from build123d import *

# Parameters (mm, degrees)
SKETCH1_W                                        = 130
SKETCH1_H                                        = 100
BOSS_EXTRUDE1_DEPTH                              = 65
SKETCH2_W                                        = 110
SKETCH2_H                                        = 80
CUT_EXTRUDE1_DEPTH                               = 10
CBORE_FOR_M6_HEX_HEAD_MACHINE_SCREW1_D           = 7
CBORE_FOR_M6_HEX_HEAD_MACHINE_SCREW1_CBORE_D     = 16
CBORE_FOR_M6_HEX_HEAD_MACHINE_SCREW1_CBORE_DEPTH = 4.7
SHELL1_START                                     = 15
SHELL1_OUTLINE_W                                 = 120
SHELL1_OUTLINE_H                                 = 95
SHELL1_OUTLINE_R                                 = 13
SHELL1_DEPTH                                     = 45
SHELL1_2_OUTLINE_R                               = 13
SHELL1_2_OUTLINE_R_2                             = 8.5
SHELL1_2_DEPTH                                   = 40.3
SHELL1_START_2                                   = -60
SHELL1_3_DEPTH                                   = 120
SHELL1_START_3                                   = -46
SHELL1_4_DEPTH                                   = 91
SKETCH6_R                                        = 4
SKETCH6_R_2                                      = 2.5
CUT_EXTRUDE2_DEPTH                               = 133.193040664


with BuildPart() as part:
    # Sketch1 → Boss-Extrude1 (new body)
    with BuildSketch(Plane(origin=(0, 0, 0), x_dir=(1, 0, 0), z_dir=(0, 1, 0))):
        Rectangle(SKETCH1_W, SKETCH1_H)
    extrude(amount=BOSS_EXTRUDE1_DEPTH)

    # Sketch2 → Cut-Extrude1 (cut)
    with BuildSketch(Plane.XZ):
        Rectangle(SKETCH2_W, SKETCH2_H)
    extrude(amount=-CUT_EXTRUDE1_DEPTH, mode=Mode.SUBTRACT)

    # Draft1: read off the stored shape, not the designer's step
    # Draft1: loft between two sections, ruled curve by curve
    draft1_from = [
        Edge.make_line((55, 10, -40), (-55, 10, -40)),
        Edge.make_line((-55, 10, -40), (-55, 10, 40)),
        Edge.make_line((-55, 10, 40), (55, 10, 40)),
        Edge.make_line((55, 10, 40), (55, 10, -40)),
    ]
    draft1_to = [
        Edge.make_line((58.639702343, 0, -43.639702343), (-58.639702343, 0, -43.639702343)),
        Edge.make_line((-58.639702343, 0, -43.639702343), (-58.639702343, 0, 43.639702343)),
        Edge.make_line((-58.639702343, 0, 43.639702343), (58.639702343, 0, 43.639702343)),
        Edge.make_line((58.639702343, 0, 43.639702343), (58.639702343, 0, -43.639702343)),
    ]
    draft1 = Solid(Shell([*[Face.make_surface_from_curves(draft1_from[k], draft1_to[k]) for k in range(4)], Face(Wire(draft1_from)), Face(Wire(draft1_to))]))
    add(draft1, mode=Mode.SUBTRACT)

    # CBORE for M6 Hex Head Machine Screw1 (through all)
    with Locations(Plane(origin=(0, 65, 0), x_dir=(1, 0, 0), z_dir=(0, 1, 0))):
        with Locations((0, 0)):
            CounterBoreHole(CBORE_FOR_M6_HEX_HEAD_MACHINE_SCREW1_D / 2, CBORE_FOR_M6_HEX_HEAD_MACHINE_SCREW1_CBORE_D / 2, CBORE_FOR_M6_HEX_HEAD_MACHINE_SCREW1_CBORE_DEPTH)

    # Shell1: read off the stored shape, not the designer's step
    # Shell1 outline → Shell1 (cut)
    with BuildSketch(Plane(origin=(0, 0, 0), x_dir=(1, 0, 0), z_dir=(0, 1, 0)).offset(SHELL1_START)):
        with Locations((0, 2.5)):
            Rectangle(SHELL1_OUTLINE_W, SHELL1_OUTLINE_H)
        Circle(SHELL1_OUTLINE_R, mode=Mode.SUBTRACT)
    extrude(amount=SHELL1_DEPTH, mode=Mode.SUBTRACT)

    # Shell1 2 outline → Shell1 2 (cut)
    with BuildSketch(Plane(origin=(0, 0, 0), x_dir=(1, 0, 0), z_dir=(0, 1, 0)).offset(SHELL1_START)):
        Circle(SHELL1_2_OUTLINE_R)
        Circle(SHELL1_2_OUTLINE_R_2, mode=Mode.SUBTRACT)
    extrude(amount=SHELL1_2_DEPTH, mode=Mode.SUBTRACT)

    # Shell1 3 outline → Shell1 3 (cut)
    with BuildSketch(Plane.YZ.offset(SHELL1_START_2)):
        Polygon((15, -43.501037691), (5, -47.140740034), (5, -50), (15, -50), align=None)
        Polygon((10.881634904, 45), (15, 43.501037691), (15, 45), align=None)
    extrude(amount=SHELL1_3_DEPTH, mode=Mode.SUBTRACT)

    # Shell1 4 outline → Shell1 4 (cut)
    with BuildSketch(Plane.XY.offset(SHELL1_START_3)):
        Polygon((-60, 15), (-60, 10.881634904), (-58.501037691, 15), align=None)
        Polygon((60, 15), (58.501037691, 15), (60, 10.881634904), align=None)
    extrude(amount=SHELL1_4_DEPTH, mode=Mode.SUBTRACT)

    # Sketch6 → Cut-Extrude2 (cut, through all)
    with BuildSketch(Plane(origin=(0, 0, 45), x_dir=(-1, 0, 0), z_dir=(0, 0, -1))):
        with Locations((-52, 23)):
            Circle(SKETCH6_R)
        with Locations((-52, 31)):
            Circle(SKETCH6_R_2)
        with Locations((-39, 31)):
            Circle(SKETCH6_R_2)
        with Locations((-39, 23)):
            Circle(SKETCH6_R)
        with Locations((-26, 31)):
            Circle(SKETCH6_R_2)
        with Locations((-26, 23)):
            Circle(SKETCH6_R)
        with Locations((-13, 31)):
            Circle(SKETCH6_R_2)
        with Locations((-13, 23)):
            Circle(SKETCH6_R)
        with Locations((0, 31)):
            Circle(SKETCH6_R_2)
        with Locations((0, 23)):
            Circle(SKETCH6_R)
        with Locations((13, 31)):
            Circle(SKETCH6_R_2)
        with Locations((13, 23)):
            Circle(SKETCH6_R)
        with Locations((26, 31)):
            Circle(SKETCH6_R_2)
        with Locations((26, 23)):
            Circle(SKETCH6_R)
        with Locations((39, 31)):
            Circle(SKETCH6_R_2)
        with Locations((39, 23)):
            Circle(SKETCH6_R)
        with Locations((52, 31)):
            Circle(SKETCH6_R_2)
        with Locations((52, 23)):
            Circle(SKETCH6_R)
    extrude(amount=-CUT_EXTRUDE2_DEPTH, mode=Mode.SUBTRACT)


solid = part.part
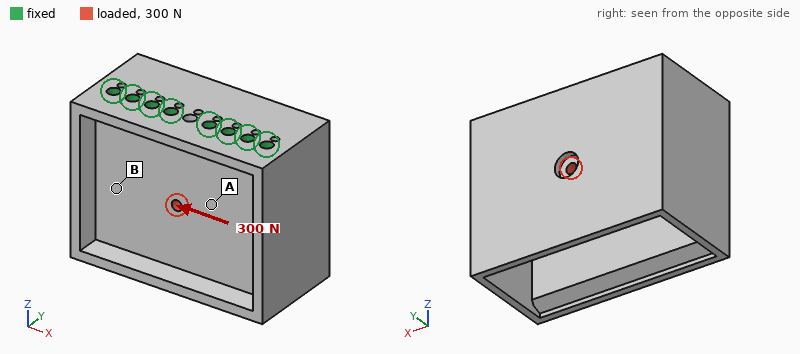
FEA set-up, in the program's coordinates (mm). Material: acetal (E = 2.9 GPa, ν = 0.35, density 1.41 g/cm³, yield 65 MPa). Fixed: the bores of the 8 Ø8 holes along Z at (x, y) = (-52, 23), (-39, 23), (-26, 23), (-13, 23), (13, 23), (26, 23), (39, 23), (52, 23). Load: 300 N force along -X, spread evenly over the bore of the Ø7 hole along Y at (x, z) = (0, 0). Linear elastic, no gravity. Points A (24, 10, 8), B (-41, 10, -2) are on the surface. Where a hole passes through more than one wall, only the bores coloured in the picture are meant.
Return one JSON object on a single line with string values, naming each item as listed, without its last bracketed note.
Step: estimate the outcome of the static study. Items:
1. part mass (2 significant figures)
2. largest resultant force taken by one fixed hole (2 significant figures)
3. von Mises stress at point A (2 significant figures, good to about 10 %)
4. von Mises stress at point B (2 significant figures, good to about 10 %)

{"part mass": "330 g", "largest resultant force taken by one fixed hole": "120 N", "von Mises stress at point A": "0.96 MPa", "von Mises stress at point B": "0.39 MPa"}
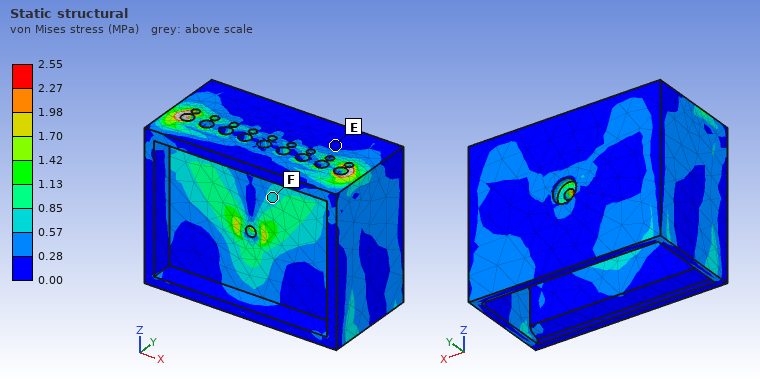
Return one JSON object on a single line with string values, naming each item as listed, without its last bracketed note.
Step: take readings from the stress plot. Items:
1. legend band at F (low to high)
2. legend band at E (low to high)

{"legend band at F": "0.57 to 0.85 MPa", "legend band at E": "0.00 to 0.28 MPa"}
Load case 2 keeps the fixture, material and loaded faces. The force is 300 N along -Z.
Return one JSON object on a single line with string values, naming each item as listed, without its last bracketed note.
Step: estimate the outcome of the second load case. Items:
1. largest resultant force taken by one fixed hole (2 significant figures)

{"largest resultant force taken by one fixed hole": "130 N"}
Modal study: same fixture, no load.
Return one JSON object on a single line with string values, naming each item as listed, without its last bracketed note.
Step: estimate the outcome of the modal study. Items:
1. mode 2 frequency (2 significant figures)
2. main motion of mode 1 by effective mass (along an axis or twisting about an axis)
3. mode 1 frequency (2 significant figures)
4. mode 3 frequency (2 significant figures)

{"mode 2 frequency": "400 Hz", "main motion of mode 1 by effective mass": "along Y", "mode 1 frequency": "170 Hz", "mode 3 frequency": "700 Hz"}
